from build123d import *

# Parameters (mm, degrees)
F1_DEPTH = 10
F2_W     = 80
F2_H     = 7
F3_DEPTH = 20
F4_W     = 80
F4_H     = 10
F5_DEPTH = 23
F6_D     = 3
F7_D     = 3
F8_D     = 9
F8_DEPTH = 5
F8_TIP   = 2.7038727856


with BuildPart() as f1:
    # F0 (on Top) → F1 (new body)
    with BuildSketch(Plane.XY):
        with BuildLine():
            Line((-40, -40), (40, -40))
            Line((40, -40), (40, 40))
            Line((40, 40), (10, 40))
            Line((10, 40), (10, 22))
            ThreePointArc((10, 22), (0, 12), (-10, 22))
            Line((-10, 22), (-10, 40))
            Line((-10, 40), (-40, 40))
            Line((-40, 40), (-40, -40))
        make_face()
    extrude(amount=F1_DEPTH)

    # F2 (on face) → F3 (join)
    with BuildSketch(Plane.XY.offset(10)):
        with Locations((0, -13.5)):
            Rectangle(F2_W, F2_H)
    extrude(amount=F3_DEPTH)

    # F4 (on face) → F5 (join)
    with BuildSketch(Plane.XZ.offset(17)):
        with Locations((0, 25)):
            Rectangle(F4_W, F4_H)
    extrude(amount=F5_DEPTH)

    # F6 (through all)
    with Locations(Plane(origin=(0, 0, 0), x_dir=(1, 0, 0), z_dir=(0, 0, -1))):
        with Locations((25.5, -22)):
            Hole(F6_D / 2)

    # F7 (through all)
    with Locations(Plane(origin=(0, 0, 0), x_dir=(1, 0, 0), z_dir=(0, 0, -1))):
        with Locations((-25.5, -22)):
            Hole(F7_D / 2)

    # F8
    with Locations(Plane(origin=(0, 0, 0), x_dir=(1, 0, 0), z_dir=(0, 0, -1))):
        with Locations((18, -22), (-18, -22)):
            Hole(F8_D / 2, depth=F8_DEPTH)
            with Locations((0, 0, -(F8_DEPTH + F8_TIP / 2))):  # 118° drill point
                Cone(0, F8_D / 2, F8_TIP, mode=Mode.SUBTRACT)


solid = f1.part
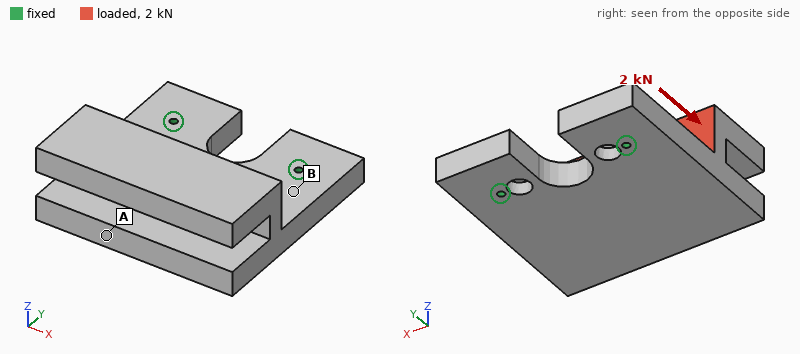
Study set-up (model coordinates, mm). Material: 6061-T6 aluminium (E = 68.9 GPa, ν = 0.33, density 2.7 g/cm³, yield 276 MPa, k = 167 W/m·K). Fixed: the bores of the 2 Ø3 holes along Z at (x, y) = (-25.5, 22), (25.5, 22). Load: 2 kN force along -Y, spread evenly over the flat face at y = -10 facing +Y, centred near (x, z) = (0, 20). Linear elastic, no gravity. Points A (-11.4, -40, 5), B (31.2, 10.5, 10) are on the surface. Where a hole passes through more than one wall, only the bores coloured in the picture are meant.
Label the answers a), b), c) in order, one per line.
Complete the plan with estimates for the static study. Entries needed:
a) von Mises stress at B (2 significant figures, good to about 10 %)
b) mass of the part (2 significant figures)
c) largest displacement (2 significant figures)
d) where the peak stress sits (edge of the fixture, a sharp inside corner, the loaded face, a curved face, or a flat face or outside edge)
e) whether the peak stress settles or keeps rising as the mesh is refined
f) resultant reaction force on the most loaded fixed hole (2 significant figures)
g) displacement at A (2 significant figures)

a) 30 MPa
b) 240 g
c) 0.20 mm
d) edge of the fixture
e) keeps rising
f) 1.0 kN
g) 0.15 mm
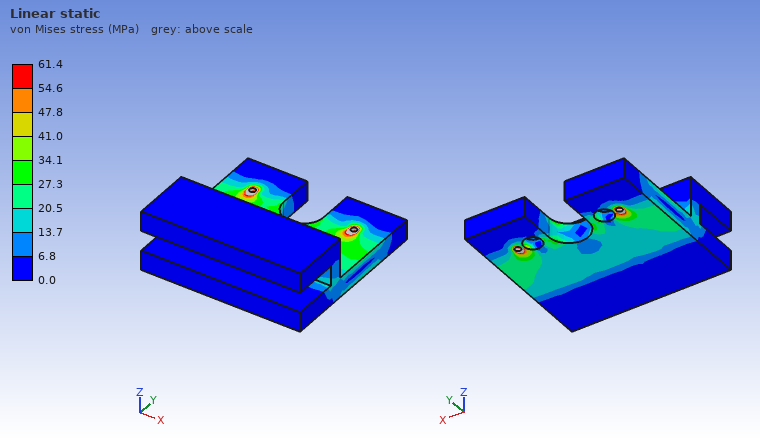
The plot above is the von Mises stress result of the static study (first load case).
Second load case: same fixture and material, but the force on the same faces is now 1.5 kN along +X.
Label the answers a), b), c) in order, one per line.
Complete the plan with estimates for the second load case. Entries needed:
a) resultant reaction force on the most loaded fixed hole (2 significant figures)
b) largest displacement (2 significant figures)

a) 1.2 kN
b) 35 µm
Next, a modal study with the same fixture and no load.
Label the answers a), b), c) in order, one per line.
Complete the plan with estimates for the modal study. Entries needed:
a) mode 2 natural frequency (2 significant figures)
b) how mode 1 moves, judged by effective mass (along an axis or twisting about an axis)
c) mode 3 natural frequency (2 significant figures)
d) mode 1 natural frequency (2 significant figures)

a) 2600 Hz
b) along Z
c) 4400 Hz
d) 1000 Hz
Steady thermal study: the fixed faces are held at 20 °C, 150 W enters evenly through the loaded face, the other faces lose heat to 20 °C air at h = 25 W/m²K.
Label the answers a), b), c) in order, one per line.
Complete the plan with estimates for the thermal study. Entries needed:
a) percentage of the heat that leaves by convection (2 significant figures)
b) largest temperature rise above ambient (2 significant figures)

a) 14 %
b) 65 K
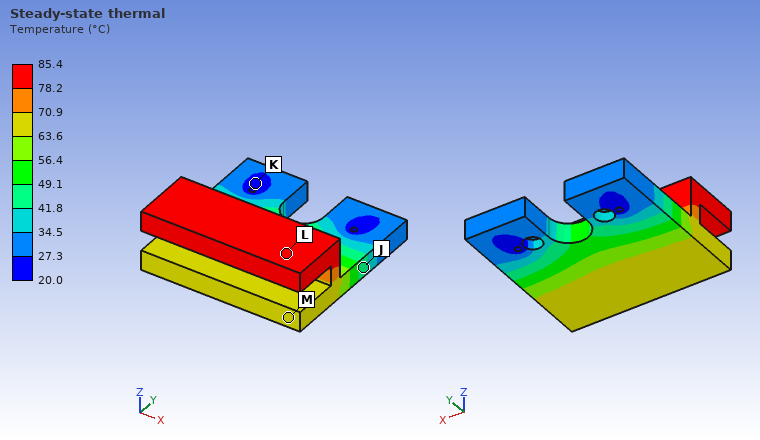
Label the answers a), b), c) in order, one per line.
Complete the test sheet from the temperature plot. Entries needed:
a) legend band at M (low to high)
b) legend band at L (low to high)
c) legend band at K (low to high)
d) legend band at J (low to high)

a) 63.6 to 70.9 °C
b) 78.2 to 85.4 °C
c) 20.0 to 27.3 °C
d) 41.8 to 49.1 °C
